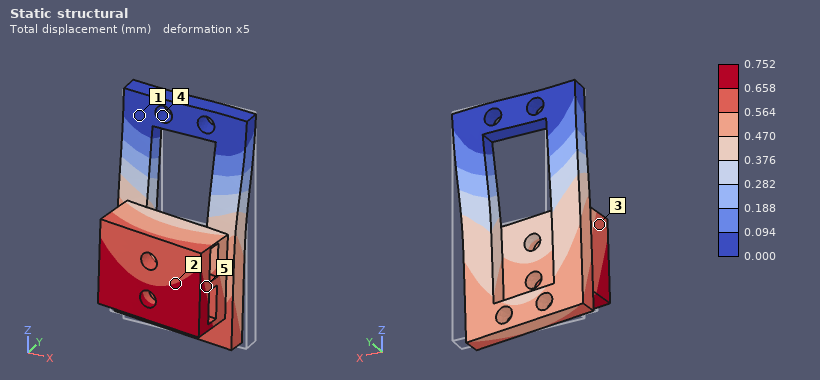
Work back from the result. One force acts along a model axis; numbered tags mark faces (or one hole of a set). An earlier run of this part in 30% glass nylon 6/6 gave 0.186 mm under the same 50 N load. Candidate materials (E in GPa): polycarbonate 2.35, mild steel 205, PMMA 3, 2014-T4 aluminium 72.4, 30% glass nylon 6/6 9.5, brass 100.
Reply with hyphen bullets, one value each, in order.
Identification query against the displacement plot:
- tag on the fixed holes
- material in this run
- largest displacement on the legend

- 4
- polycarbonate
- 0.752 mm
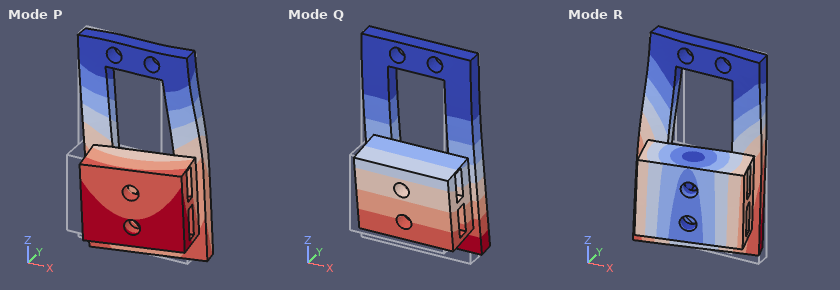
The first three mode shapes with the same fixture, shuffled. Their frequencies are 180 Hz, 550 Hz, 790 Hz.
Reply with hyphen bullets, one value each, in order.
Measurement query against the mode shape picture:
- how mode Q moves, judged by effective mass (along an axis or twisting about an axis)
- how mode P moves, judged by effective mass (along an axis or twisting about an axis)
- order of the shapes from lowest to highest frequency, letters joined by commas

- along Y
- along X
- Q, P, R
